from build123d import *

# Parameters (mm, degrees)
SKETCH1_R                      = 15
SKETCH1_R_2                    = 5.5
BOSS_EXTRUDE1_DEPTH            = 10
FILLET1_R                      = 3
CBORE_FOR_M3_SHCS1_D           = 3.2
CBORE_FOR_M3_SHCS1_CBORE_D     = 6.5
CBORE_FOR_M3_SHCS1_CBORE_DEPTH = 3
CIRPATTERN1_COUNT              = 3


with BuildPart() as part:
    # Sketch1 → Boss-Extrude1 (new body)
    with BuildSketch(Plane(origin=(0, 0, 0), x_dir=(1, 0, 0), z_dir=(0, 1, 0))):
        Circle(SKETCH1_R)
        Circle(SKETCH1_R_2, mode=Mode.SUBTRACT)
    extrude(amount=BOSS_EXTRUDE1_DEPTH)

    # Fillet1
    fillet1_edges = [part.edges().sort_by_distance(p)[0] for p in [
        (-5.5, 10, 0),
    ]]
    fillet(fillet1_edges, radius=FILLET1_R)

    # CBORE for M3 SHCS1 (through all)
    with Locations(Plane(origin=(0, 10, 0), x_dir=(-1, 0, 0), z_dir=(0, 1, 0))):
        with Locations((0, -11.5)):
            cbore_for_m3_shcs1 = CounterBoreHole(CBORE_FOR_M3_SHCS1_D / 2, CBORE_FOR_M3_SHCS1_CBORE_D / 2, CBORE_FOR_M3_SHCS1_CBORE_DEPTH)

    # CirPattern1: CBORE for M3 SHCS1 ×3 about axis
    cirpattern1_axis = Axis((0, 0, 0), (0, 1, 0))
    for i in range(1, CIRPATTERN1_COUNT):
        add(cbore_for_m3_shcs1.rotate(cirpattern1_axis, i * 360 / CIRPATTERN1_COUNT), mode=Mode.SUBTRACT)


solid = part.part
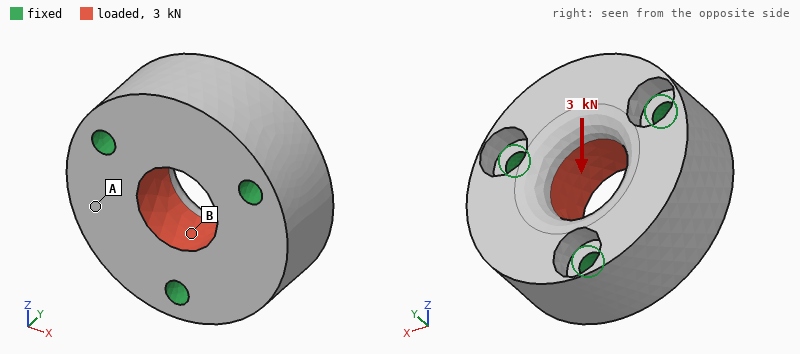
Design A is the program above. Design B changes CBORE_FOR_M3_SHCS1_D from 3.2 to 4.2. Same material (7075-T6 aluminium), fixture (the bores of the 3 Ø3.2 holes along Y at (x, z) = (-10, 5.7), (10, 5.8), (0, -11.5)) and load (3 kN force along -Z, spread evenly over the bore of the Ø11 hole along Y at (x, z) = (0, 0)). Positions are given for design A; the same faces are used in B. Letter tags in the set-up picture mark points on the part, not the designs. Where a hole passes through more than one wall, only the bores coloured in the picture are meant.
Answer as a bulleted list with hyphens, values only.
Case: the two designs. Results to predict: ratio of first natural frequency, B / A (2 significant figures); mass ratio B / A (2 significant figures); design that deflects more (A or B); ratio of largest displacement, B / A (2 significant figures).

- 1.1
- 0.98
- A
- 0.91
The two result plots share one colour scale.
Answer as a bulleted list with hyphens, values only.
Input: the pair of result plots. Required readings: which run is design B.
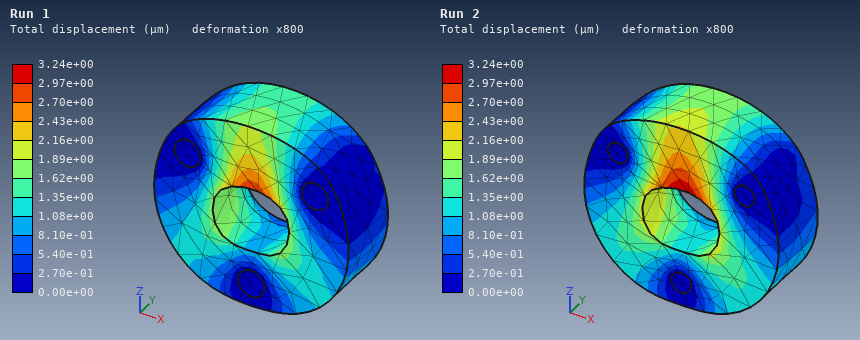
- Run 1
